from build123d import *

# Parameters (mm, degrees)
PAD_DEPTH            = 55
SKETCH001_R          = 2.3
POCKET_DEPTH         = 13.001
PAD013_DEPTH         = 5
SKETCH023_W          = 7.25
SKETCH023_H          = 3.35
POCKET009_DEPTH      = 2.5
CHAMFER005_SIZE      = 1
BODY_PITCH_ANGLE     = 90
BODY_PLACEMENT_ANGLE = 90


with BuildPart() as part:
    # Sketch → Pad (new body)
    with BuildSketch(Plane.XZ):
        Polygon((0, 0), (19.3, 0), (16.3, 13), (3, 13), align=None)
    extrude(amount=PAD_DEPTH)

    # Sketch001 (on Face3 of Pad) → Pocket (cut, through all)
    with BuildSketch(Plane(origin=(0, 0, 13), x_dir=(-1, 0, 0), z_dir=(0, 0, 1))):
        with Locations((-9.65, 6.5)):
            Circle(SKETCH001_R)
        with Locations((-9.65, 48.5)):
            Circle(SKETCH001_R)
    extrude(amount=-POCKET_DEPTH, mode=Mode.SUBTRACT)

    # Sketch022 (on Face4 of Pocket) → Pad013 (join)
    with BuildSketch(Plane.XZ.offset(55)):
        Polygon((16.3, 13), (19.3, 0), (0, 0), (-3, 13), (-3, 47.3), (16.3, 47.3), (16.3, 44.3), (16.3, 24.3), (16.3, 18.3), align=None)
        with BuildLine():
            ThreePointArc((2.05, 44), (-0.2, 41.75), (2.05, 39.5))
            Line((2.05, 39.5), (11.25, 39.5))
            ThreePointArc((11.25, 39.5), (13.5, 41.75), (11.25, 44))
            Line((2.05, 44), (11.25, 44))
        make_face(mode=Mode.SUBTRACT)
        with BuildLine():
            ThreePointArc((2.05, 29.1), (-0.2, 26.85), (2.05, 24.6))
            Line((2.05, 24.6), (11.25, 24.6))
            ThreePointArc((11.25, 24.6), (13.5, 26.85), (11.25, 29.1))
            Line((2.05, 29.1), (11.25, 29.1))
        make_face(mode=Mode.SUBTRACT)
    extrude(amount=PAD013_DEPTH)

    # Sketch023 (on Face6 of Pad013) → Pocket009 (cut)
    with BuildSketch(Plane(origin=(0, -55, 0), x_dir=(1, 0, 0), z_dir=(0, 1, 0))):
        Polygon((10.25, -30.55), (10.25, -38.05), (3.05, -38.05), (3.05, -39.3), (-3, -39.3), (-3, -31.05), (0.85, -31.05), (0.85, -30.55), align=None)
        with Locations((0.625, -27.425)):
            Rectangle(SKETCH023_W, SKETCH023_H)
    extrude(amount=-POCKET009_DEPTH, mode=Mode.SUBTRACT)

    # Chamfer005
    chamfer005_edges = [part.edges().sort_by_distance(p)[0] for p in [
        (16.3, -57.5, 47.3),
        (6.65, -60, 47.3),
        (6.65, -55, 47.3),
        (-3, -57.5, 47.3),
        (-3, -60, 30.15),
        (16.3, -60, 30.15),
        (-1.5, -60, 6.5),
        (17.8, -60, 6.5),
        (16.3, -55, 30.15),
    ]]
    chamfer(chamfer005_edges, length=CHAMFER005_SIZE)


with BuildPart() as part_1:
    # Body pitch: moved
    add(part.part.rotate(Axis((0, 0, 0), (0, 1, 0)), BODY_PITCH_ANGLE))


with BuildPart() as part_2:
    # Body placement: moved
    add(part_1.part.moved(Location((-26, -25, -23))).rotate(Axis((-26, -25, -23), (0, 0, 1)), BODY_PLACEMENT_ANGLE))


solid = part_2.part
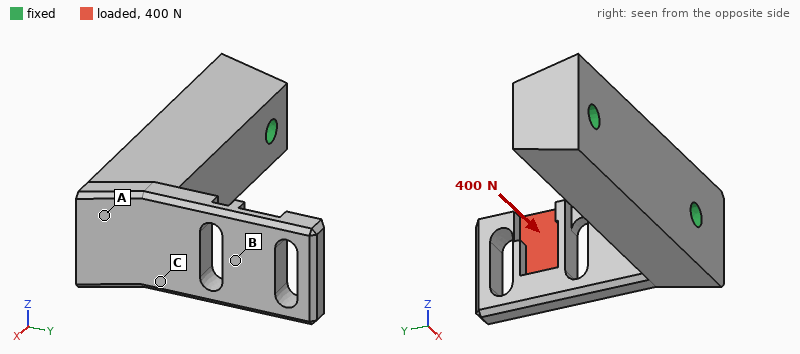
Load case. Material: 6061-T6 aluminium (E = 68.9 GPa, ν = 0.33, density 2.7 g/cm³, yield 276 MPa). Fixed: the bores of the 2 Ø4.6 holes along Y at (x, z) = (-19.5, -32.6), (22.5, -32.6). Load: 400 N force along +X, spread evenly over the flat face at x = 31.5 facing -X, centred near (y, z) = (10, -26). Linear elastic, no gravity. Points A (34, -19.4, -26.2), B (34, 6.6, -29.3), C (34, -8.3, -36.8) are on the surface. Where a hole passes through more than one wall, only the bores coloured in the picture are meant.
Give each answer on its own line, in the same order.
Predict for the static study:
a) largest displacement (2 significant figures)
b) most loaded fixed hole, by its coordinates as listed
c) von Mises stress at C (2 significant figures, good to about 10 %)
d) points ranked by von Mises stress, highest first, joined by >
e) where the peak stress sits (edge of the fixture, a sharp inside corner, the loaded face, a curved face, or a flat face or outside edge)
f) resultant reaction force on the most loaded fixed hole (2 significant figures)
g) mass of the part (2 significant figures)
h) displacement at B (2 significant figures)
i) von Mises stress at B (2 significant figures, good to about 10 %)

0.59 mm
(22.5, -32.6)
110 MPa
C > B > A
a curved face
420 N
40 g
0.21 mm
69 MPa
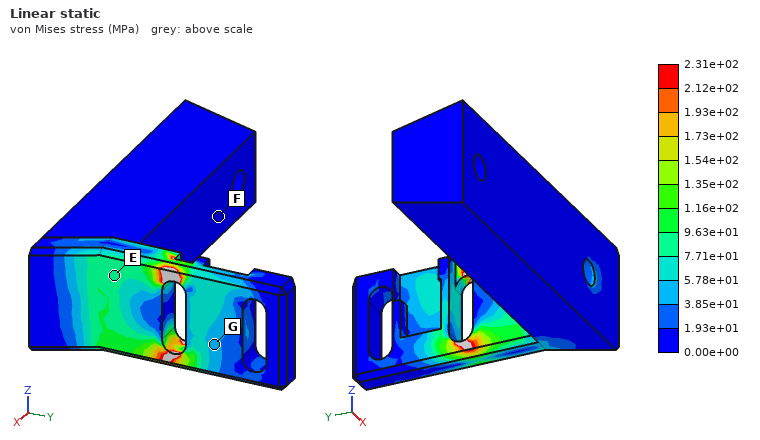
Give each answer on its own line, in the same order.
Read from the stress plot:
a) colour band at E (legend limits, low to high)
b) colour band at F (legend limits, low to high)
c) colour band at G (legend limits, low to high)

7.71e+01 to 9.63e+01 MPa
0.00e+00 to 1.93e+01 MPa
3.85e+01 to 5.78e+01 MPa
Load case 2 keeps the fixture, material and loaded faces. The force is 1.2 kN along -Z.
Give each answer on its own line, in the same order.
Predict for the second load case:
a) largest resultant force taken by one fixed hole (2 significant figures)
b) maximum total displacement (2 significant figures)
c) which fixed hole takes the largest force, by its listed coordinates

1.3 kN
0.24 mm
(22.5, -32.6)
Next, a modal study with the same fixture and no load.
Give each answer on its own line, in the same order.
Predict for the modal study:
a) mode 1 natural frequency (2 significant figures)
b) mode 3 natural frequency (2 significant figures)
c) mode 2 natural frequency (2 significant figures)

2500 Hz
8100 Hz
6400 Hz
